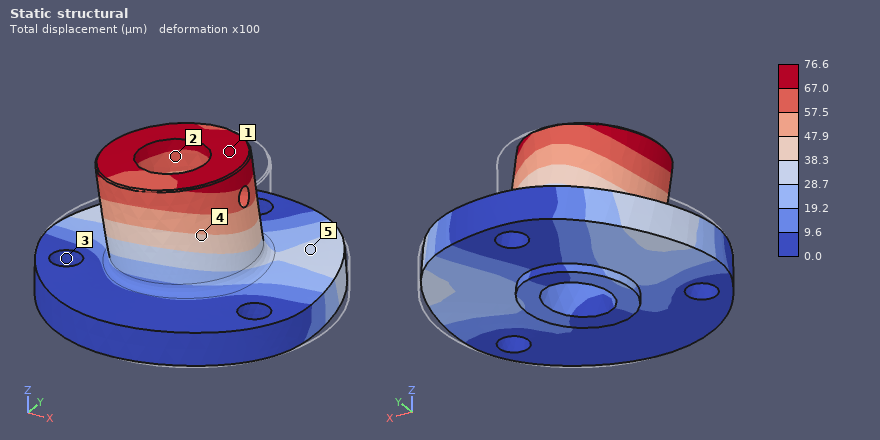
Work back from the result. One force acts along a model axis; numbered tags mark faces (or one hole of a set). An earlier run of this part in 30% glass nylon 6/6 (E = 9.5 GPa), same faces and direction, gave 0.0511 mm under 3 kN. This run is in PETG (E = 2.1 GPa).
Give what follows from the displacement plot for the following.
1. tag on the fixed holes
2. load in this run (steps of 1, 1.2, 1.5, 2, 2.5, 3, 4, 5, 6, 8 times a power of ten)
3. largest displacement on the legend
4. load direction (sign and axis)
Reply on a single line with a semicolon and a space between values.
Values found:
3; 1 kN; 76.6 µm; -X
